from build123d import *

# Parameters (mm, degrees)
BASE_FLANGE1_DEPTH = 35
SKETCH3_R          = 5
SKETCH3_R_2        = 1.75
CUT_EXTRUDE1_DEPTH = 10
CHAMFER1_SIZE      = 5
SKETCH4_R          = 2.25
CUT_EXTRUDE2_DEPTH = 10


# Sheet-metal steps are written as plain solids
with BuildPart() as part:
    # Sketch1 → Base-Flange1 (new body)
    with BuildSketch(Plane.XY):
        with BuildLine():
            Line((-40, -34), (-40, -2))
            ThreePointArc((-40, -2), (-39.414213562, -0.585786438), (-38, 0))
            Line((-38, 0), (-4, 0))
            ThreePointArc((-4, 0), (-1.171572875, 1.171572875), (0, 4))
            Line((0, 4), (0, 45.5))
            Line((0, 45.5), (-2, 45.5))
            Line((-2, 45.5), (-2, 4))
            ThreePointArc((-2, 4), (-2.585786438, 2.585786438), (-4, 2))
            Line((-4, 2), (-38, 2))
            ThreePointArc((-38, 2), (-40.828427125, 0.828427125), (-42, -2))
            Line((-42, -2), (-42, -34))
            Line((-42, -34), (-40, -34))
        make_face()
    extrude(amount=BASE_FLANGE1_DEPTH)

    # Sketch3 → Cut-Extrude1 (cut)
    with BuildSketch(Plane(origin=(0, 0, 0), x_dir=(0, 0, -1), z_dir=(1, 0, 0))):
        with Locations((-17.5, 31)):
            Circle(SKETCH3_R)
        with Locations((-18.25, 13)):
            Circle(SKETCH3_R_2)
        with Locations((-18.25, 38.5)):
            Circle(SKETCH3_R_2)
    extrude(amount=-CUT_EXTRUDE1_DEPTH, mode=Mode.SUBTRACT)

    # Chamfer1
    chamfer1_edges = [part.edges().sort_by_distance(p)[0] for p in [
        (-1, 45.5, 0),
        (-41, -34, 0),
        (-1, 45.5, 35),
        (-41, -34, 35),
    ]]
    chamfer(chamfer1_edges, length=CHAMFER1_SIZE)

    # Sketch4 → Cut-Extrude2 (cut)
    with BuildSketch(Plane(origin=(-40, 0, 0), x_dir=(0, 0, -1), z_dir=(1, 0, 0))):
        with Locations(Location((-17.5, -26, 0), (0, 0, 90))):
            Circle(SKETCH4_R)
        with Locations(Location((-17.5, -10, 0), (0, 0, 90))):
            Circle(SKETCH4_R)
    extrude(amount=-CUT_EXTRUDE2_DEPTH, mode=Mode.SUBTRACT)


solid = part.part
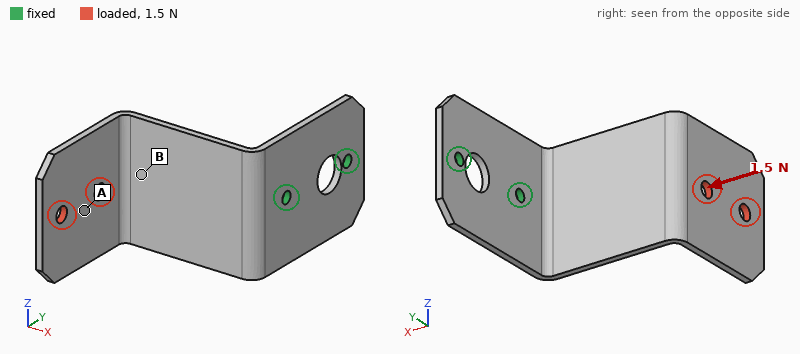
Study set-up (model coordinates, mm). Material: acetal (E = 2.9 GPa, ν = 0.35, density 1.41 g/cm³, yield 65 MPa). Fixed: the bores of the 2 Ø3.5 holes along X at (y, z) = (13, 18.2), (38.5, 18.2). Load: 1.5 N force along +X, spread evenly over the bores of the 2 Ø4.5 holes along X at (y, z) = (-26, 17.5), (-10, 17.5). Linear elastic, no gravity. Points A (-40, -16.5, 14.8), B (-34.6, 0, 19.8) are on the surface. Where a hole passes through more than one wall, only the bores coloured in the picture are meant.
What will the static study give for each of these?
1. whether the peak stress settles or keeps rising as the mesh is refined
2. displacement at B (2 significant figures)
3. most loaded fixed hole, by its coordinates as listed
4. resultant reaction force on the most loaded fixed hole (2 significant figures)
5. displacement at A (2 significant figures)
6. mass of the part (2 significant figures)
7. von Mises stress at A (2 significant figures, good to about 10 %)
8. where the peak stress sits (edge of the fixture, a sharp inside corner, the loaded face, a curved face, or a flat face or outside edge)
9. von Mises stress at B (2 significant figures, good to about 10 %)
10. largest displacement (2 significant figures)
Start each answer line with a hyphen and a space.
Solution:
- keeps rising
- 0.45 mm
- (13, 18.2)
- 2.0 N
- 0.73 mm
- 11 g
- 0.32 MPa
- edge of the fixture
- 1.2 MPa
- 1.1 mm
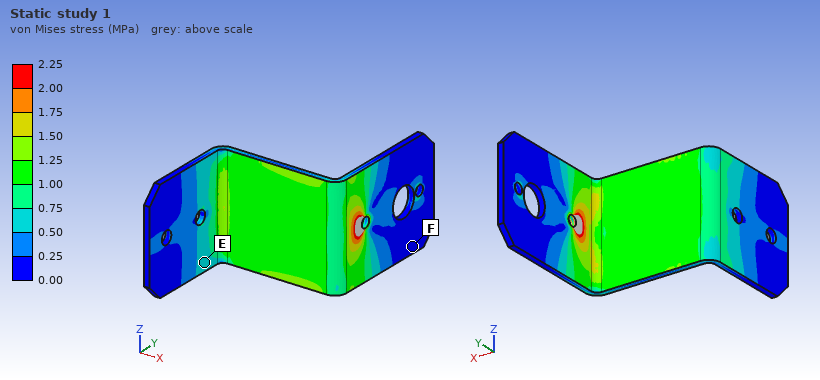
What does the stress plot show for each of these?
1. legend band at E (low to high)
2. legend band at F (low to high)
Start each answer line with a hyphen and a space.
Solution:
- 0.50 to 0.75 MPa
- 0.00 to 0.25 MPa
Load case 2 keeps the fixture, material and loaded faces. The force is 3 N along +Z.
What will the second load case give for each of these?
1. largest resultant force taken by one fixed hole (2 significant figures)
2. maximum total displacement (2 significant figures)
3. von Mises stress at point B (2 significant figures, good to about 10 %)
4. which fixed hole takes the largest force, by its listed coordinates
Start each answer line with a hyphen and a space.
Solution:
- 6.0 N
- 0.93 mm
- 1.7 MPa
- (13, 18.2)
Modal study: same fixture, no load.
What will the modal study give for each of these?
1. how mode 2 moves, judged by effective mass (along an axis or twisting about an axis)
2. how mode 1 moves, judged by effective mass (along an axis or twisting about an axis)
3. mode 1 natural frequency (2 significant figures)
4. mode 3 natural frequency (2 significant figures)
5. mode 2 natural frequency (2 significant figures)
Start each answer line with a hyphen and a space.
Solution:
- along Z
- along Y
- 86 Hz
- 280 Hz
- 170 Hz
